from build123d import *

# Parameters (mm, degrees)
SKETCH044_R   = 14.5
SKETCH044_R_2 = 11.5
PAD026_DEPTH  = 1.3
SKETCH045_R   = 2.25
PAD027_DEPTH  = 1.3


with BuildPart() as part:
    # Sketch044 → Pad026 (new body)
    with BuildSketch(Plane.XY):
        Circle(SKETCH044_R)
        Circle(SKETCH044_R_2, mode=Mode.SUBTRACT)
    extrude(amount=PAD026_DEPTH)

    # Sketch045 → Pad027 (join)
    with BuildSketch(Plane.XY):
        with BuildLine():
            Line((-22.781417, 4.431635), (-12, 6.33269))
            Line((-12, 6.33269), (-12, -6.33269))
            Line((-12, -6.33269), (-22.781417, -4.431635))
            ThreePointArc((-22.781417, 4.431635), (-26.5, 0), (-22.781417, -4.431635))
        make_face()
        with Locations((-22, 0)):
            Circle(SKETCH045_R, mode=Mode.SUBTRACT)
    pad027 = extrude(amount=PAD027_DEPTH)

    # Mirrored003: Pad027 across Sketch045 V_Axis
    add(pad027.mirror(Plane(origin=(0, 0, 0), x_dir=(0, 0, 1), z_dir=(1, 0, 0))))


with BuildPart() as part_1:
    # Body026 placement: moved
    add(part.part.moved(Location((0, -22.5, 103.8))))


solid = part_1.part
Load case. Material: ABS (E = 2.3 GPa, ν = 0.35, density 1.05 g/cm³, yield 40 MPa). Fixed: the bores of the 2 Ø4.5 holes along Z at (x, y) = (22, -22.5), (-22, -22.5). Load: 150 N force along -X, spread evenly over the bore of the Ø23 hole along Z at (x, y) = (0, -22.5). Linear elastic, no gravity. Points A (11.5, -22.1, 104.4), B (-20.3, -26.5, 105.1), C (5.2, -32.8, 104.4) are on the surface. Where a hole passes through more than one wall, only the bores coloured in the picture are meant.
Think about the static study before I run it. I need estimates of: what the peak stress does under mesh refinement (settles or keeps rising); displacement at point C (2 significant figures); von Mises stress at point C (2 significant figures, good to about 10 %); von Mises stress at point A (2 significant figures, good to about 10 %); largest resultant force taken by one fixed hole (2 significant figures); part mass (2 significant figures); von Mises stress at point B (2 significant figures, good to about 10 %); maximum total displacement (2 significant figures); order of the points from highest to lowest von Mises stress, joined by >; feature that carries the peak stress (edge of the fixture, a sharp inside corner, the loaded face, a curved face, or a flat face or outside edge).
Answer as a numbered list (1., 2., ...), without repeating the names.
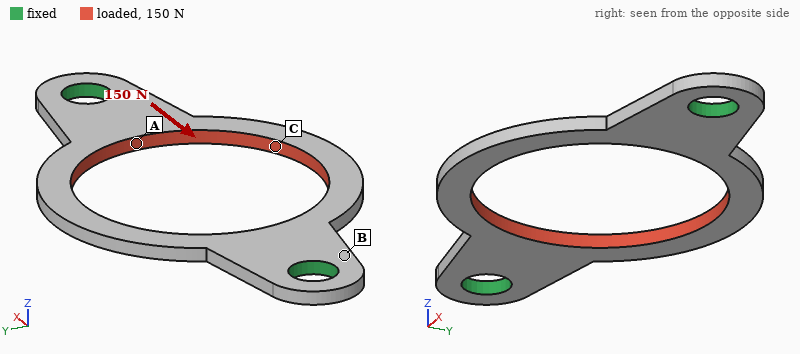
1. keeps rising
2. 0.19 mm
3. 23 MPa
4. 11 MPa
5. 75 N
6. 0.61 g
7. 4.5 MPa
8. 0.19 mm
9. C > A > B
10. a sharp inside corner
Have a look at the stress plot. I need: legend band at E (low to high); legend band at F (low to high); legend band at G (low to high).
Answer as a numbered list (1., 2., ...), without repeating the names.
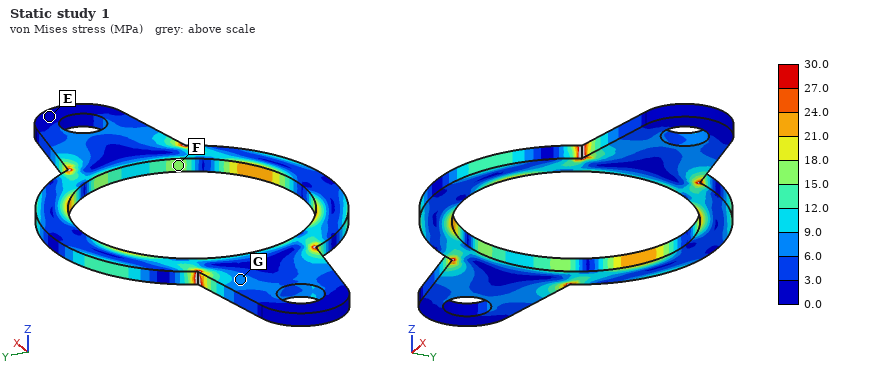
1. 0.0 to 3.0 MPa
2. 15.0 to 18.0 MPa
3. 6.0 to 9.0 MPa
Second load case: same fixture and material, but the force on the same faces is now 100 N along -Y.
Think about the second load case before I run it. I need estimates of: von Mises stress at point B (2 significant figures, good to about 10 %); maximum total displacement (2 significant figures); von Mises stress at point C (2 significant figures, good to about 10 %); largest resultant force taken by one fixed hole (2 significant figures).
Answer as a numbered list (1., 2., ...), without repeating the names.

1. 6.6 MPa
2. 99 µm
3. 6.5 MPa
4. 50 N
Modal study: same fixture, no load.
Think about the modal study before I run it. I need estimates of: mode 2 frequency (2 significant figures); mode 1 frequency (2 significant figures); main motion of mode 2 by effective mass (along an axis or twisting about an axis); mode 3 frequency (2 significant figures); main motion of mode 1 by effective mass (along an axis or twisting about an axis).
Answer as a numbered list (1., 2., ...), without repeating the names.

1. 1000 Hz
2. 940 Hz
3. along Z
4. 2600 Hz
5. twisting about X
